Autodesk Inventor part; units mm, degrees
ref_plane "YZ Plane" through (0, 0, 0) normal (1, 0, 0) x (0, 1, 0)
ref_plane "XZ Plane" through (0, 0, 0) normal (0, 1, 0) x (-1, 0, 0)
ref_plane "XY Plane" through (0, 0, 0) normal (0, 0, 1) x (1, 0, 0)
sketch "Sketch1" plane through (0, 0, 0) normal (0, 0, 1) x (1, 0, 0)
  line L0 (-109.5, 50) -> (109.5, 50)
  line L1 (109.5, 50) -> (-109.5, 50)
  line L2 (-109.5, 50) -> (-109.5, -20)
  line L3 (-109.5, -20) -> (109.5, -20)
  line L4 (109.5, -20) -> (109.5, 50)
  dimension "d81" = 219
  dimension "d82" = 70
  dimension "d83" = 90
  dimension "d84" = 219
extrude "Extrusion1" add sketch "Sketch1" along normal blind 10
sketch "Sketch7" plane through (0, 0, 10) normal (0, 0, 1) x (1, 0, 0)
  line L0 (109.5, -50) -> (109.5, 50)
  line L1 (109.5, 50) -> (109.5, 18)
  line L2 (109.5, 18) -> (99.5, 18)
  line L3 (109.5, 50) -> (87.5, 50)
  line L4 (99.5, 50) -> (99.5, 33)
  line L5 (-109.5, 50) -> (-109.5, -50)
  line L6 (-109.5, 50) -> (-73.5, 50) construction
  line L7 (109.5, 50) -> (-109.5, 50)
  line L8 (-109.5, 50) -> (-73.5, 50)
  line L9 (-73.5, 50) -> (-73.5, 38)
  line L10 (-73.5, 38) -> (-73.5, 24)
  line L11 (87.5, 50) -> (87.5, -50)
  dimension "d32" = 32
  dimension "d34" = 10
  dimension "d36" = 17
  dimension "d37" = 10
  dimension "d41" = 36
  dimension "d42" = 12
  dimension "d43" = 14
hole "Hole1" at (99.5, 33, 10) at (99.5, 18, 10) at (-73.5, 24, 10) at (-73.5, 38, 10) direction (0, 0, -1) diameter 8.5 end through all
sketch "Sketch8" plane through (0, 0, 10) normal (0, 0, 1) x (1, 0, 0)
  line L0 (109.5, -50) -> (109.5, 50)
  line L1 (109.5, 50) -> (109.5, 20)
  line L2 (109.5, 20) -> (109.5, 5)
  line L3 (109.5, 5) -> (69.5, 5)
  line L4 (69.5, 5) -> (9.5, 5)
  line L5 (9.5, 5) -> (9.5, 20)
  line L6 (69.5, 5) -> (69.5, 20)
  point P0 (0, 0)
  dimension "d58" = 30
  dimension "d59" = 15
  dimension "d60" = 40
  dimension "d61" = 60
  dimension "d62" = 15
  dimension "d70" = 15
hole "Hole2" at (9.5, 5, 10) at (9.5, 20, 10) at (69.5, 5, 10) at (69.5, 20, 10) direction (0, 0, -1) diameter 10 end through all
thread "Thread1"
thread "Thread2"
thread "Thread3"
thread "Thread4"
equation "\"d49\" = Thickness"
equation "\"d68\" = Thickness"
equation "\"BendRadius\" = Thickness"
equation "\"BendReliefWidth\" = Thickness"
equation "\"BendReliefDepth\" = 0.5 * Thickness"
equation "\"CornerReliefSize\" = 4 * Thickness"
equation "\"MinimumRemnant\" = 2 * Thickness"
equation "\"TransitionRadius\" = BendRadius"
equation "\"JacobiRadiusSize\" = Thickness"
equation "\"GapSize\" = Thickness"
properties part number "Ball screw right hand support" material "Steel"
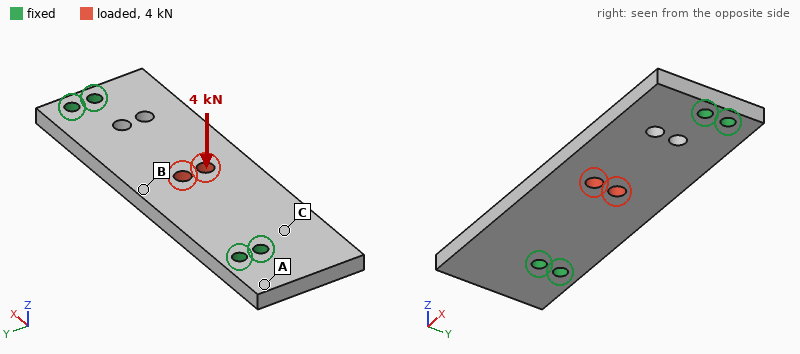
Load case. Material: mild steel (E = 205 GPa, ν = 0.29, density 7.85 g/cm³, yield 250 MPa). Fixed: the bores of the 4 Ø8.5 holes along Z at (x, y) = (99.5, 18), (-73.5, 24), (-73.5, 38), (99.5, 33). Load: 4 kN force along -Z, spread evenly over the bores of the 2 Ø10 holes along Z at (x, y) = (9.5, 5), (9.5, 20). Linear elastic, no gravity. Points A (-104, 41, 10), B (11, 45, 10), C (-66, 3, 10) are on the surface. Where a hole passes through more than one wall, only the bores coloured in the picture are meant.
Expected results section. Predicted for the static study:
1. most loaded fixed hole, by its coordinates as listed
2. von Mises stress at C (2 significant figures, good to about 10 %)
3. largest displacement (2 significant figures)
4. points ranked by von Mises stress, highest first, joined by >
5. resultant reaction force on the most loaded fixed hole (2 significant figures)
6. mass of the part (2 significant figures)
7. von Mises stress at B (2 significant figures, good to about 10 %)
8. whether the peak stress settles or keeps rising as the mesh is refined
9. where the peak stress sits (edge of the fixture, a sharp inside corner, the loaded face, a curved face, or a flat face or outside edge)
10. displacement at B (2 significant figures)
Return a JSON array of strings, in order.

["(-73.5, 24)", "42 MPa", "0.13 mm", "B > C > A", "2.2 kN", "1.2 kg", "67 MPa", "keeps rising", "edge of the fixture", "0.088 mm"]
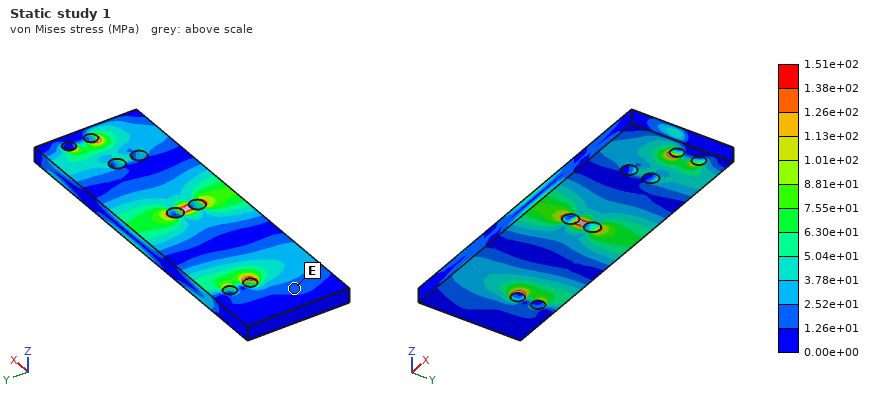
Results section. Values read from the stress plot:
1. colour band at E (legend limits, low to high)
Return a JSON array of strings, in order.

["1.26e+01 to 2.52e+01 MPa"]
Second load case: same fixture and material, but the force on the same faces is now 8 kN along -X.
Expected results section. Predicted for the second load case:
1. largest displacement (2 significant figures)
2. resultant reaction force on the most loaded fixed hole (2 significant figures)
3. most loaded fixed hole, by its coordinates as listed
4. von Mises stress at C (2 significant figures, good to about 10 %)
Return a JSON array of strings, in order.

["4.3 µm", "3.1 kN", "(-73.5, 24)", "3.6 MPa"]
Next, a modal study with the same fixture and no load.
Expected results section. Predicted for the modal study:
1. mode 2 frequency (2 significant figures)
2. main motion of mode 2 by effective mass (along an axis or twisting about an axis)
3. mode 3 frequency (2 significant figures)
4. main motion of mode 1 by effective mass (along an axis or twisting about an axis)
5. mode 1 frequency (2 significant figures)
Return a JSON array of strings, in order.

["2600 Hz", "twisting about X", "3700 Hz", "along Z", "1600 Hz"]
